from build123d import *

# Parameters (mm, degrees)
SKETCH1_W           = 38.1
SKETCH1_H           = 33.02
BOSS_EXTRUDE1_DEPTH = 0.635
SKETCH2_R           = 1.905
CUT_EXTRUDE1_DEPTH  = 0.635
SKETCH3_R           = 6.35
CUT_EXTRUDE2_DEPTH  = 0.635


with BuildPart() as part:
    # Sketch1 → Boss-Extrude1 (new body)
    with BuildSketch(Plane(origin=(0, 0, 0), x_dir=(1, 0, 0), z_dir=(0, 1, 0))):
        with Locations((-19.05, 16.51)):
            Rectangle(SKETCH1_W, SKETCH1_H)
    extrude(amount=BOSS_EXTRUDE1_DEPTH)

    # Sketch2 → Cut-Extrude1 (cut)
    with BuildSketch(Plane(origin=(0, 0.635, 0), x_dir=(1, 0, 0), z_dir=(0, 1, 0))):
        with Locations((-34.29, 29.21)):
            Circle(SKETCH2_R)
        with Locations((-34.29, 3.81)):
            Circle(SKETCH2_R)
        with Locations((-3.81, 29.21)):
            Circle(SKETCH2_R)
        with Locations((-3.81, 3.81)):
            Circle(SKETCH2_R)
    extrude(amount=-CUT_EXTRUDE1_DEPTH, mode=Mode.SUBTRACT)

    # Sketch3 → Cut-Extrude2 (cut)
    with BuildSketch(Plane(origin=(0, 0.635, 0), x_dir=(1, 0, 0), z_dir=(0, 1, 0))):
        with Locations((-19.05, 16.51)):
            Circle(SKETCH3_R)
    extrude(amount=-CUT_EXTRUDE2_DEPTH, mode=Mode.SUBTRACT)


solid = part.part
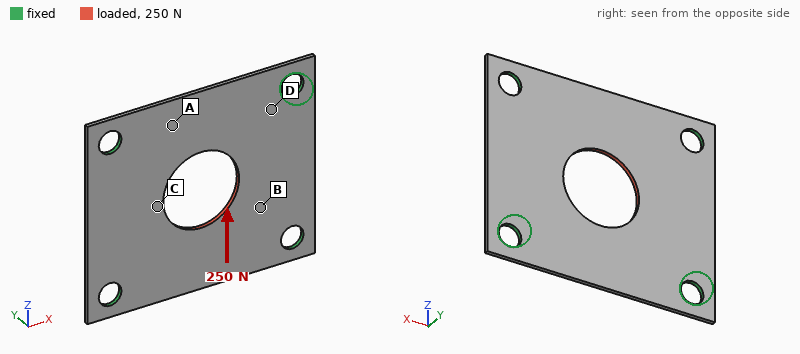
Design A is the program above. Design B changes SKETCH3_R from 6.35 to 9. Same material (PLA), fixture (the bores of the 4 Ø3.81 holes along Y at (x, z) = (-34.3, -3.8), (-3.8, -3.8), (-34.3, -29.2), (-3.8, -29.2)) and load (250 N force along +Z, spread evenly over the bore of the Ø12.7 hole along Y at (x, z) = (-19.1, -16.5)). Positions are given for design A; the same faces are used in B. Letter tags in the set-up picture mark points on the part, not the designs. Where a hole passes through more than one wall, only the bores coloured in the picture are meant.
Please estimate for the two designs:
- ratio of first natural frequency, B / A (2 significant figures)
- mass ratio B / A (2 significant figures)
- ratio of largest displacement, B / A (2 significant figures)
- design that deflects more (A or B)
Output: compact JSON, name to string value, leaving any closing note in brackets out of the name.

{"ratio of first natural frequency, B / A": "1.2", "mass ratio B / A": "0.88", "ratio of largest displacement, B / A": "1.1", "design that deflects more": "B"}
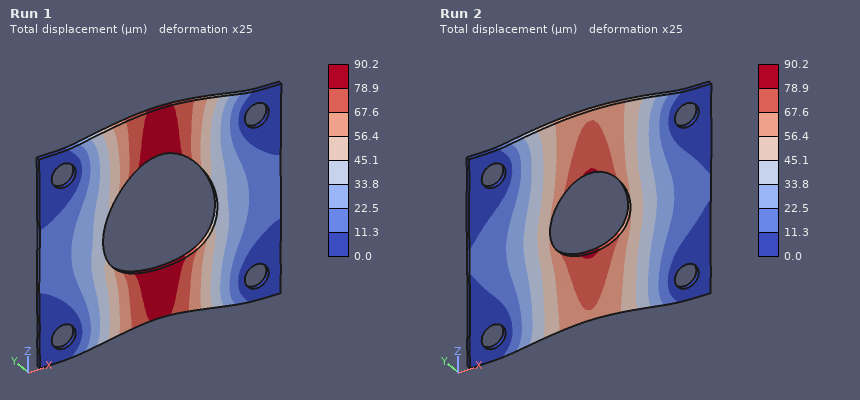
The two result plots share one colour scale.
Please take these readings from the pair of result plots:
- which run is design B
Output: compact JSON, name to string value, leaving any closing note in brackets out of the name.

{"which run is design B": "Run 1"}
